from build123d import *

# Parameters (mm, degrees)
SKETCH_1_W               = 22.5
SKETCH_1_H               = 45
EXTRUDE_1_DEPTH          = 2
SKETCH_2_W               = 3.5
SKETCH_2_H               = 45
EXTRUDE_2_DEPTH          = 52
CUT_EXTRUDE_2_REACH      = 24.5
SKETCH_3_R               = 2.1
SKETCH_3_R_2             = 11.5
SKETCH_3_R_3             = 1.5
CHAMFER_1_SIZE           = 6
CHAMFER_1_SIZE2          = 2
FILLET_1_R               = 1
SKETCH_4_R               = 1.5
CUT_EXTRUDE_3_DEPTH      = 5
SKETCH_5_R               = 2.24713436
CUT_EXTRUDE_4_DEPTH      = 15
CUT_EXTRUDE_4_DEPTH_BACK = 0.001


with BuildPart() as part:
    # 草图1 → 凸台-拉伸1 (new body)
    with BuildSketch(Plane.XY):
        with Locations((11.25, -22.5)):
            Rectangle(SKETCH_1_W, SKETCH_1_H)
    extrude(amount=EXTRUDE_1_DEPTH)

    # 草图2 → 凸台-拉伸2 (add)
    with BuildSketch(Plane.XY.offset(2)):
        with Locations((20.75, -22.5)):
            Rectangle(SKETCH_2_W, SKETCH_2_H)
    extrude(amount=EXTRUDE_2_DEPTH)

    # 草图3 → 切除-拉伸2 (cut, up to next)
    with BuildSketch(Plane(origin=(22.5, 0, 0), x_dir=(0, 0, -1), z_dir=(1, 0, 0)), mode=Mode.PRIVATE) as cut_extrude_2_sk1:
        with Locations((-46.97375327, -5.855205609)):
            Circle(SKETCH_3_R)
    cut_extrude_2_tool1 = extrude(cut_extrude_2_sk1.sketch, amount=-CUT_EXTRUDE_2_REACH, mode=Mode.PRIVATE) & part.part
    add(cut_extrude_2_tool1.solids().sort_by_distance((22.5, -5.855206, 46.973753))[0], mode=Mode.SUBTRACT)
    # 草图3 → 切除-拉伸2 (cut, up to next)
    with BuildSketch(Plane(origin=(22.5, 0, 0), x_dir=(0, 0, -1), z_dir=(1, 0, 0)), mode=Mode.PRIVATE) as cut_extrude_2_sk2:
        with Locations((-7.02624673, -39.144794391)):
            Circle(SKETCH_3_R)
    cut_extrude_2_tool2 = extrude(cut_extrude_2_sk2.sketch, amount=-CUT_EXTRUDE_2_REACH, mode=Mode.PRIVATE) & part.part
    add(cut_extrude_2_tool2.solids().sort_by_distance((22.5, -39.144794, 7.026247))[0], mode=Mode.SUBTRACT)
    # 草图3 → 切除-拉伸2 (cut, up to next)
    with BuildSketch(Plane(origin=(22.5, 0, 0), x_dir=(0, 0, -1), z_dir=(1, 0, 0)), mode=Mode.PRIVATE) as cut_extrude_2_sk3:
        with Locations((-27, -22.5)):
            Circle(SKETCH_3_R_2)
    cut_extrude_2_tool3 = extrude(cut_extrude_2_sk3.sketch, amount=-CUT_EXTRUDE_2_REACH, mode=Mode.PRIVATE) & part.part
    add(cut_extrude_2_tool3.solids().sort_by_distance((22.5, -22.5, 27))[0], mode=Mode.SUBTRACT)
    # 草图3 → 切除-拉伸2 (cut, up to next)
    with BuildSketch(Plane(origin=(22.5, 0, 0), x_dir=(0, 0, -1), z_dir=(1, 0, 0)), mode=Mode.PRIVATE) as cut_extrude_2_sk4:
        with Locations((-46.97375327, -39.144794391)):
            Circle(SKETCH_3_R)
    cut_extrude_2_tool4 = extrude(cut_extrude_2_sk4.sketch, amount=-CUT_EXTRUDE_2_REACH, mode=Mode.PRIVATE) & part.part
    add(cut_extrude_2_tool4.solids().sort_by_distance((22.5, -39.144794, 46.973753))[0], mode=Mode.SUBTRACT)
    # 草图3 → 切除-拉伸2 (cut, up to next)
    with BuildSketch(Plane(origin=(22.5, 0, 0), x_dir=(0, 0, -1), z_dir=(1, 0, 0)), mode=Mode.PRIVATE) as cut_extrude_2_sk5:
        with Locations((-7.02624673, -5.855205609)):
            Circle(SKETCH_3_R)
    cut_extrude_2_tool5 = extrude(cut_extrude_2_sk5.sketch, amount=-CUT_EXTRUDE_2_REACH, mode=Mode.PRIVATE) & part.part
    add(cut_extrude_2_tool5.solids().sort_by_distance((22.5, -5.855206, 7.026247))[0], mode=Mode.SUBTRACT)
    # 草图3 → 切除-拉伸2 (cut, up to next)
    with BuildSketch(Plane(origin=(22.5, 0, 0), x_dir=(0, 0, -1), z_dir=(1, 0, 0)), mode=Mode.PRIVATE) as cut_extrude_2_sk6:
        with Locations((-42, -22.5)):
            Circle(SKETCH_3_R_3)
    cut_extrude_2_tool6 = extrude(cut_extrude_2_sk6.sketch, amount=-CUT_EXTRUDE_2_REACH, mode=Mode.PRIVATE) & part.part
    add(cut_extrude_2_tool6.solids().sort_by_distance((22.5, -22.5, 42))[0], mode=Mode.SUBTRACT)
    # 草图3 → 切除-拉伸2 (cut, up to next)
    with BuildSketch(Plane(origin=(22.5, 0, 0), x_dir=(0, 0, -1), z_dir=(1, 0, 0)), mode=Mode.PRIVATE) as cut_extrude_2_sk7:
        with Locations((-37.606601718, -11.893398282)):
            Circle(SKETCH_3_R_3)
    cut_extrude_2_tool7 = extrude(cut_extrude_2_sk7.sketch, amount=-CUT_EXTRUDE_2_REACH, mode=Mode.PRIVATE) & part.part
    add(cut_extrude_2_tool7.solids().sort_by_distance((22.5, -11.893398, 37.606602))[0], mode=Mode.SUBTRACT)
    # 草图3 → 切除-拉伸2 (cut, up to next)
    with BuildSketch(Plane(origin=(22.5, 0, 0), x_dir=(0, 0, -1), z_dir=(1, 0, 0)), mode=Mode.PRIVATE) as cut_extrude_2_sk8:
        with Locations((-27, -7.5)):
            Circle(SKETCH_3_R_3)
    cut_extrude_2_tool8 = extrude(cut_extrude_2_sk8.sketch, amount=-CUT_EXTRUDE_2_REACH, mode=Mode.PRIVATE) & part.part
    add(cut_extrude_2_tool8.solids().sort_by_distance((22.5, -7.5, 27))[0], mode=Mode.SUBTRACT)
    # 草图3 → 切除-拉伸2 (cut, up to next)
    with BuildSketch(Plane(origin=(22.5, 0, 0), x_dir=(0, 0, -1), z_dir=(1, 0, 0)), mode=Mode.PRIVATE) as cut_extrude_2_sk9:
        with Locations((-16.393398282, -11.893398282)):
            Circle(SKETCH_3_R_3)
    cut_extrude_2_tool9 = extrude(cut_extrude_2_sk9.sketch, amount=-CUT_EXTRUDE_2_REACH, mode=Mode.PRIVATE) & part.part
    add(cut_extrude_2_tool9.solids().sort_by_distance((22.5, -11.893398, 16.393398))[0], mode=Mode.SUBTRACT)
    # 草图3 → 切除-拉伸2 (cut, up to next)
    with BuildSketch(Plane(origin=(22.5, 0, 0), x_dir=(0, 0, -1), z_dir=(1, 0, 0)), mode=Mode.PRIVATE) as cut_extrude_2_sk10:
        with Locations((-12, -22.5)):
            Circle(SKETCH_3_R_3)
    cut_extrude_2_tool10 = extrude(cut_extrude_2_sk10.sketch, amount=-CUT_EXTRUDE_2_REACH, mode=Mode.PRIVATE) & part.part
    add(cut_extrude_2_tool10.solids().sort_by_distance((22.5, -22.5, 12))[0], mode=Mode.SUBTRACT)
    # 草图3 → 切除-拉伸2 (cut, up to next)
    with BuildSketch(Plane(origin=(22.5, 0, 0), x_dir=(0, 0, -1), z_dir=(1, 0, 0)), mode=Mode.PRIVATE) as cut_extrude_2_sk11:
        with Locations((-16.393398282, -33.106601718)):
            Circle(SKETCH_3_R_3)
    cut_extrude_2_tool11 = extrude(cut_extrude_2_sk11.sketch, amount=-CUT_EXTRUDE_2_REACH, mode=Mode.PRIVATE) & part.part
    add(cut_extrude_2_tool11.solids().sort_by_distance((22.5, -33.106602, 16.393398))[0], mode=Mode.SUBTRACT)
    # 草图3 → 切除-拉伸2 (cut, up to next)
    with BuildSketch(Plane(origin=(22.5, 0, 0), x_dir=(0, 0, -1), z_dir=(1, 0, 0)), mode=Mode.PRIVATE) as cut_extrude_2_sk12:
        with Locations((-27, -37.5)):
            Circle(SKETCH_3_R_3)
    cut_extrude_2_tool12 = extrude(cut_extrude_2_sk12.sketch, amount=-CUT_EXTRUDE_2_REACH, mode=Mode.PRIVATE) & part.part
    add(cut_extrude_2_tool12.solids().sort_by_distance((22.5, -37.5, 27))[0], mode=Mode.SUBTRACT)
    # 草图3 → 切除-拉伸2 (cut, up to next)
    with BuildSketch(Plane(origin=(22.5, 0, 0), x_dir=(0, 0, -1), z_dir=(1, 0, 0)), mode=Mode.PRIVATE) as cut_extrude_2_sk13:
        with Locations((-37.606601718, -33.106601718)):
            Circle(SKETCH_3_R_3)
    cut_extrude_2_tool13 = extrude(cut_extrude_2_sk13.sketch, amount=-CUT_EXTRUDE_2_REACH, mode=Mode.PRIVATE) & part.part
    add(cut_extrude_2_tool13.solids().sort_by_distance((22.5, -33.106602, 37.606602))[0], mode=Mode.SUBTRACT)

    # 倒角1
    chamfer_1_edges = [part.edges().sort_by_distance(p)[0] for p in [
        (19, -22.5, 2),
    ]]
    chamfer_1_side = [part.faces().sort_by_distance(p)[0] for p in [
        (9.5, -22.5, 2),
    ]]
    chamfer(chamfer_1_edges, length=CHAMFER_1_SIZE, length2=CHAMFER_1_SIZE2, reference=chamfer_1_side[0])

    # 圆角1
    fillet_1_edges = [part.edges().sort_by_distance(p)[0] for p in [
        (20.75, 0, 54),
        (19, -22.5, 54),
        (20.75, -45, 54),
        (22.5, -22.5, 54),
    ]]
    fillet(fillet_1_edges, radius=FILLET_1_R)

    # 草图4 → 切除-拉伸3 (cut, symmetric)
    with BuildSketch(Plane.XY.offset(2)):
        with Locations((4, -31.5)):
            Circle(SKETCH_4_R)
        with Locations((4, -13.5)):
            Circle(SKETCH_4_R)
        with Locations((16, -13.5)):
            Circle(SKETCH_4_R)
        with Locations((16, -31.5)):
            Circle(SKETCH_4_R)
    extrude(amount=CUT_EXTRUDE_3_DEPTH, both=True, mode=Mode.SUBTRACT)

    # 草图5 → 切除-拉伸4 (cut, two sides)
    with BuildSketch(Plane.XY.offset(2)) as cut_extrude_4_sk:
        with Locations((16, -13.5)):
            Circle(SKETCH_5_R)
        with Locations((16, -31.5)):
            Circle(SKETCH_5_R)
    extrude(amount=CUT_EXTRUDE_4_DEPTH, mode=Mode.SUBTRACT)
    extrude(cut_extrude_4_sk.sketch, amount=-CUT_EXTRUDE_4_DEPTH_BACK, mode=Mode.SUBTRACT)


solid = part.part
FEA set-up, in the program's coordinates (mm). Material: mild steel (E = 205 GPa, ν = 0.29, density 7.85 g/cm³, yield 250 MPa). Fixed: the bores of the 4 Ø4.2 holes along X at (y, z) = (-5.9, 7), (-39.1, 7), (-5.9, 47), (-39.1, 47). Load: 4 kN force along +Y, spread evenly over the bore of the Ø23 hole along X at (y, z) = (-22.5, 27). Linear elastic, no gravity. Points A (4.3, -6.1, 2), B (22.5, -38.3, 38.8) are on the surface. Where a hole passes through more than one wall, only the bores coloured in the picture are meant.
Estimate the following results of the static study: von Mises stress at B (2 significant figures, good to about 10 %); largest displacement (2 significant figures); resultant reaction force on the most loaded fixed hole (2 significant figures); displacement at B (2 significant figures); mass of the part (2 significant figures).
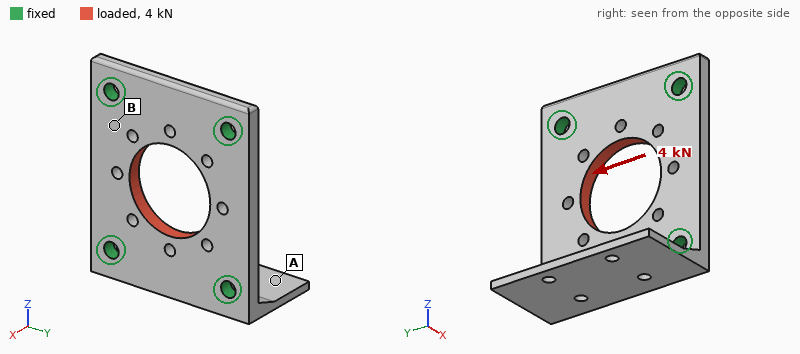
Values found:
25 MPa
4.7 µm
1.1 kN
2.0 µm
67 g
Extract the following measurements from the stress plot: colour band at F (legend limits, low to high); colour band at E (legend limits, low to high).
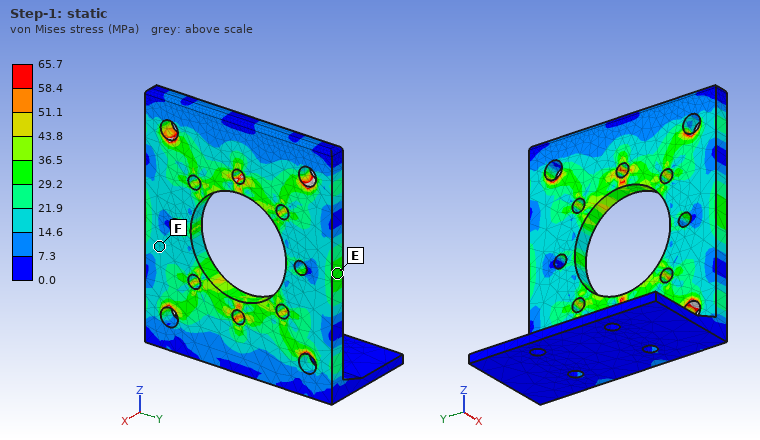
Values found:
14.6 to 21.9 MPa
29.2 to 36.5 MPa
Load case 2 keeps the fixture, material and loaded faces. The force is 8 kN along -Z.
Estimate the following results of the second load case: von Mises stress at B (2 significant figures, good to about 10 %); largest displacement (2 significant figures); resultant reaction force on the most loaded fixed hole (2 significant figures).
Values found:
42 MPa
5.9 µm
2.1 kN
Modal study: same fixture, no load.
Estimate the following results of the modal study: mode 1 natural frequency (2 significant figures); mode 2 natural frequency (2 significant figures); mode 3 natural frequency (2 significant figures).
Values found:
5200 Hz
7200 Hz
12 kHz
